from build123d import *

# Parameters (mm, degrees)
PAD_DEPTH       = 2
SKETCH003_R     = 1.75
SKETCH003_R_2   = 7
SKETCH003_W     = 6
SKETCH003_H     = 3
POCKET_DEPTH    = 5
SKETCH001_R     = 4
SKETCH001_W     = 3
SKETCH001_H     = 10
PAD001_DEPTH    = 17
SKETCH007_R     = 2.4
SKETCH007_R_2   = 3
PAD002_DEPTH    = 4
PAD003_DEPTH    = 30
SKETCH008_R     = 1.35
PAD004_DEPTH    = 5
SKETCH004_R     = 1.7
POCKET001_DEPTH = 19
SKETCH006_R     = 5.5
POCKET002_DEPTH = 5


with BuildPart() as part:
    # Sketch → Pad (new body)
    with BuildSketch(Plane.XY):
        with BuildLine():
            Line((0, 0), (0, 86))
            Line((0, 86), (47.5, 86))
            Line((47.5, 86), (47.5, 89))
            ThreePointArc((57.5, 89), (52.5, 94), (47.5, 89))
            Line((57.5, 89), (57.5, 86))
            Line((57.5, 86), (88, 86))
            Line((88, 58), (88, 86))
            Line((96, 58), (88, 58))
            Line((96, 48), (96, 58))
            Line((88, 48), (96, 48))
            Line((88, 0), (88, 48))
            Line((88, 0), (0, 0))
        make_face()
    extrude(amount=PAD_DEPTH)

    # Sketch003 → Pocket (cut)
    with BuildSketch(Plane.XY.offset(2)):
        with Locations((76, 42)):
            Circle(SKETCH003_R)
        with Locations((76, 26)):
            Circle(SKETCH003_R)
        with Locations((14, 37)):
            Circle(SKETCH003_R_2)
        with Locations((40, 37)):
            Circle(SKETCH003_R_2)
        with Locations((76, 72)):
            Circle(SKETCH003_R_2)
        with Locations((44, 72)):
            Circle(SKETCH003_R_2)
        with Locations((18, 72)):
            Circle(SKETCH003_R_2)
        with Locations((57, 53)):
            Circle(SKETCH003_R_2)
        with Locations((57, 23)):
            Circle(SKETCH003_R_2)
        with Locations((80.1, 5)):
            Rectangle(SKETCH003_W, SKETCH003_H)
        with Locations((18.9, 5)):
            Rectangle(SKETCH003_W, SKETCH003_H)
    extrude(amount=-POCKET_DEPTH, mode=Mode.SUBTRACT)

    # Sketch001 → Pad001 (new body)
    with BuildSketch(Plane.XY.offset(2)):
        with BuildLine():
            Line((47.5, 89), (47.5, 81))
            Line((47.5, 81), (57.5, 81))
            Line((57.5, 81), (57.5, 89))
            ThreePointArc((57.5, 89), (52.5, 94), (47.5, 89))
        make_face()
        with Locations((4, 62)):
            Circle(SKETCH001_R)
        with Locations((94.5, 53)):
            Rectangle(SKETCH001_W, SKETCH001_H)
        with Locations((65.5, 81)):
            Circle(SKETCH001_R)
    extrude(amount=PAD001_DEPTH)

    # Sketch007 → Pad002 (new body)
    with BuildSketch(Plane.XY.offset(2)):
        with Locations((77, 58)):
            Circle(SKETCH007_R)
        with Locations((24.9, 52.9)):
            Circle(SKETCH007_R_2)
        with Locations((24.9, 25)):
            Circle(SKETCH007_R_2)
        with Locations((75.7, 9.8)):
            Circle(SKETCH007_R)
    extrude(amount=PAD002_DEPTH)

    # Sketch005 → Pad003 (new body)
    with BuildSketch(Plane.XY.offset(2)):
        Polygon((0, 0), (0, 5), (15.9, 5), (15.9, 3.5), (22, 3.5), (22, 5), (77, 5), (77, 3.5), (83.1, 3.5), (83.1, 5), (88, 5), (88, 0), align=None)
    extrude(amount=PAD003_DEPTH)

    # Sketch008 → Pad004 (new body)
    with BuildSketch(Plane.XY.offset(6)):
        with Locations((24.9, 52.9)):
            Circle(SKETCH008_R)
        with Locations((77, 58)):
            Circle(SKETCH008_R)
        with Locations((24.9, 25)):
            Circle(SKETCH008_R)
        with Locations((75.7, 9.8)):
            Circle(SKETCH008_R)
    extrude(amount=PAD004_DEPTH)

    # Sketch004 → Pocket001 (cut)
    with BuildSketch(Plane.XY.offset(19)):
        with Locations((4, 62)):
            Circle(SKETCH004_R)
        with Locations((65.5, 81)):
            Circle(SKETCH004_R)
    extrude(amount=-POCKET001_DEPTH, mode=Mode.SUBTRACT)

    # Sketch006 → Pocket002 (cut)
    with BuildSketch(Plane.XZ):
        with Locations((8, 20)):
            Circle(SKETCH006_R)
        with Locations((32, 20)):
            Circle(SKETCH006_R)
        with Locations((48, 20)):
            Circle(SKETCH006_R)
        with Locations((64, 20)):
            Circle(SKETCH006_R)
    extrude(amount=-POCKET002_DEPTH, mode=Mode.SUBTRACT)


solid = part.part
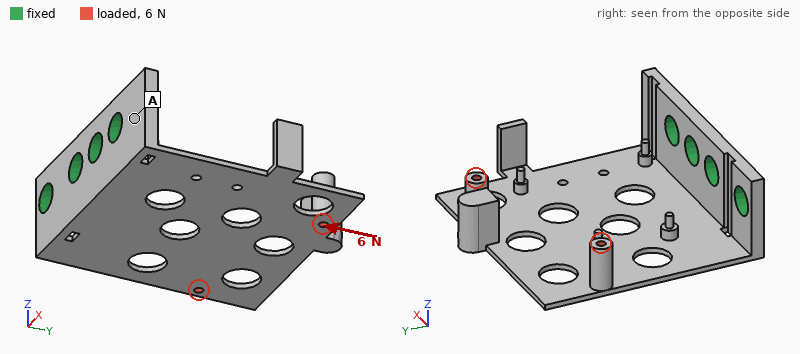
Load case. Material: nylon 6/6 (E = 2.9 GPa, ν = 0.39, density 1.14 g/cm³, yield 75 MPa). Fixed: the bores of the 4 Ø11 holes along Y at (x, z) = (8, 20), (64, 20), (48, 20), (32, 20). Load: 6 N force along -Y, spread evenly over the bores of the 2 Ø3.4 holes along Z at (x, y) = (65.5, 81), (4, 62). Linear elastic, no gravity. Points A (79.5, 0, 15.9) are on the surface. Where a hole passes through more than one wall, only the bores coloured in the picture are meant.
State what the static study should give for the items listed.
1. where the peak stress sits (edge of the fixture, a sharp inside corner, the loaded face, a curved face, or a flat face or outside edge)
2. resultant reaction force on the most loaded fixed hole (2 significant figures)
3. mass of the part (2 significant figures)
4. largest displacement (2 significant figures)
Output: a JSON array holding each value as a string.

["a curved face", "1.9 N", "32 g", "1.4 mm"]
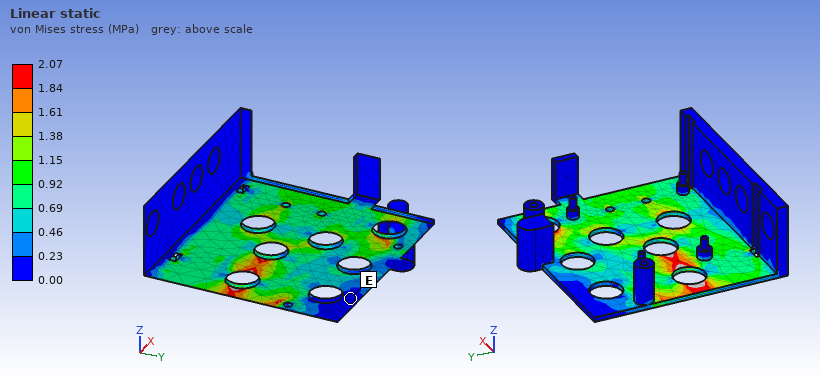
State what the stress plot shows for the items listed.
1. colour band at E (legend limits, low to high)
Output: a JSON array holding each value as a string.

["0.00 to 0.23 MPa"]
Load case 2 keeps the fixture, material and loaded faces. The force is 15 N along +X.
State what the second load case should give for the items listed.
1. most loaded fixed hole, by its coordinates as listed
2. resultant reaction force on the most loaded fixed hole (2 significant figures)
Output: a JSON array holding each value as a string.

["(64, 20)", "18 N"]
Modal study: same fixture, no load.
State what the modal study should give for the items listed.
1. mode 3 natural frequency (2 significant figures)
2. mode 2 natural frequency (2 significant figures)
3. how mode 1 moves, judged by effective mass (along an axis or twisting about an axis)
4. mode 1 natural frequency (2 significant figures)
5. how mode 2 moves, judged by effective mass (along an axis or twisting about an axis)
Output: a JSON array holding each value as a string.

["250 Hz", "130 Hz", "along Z", "53 Hz", "twisting about Y"]
